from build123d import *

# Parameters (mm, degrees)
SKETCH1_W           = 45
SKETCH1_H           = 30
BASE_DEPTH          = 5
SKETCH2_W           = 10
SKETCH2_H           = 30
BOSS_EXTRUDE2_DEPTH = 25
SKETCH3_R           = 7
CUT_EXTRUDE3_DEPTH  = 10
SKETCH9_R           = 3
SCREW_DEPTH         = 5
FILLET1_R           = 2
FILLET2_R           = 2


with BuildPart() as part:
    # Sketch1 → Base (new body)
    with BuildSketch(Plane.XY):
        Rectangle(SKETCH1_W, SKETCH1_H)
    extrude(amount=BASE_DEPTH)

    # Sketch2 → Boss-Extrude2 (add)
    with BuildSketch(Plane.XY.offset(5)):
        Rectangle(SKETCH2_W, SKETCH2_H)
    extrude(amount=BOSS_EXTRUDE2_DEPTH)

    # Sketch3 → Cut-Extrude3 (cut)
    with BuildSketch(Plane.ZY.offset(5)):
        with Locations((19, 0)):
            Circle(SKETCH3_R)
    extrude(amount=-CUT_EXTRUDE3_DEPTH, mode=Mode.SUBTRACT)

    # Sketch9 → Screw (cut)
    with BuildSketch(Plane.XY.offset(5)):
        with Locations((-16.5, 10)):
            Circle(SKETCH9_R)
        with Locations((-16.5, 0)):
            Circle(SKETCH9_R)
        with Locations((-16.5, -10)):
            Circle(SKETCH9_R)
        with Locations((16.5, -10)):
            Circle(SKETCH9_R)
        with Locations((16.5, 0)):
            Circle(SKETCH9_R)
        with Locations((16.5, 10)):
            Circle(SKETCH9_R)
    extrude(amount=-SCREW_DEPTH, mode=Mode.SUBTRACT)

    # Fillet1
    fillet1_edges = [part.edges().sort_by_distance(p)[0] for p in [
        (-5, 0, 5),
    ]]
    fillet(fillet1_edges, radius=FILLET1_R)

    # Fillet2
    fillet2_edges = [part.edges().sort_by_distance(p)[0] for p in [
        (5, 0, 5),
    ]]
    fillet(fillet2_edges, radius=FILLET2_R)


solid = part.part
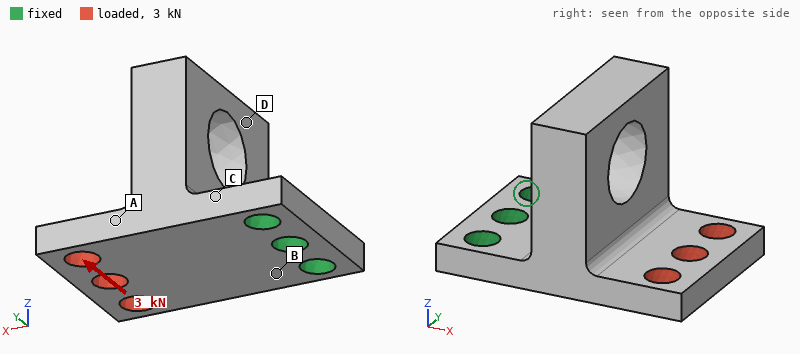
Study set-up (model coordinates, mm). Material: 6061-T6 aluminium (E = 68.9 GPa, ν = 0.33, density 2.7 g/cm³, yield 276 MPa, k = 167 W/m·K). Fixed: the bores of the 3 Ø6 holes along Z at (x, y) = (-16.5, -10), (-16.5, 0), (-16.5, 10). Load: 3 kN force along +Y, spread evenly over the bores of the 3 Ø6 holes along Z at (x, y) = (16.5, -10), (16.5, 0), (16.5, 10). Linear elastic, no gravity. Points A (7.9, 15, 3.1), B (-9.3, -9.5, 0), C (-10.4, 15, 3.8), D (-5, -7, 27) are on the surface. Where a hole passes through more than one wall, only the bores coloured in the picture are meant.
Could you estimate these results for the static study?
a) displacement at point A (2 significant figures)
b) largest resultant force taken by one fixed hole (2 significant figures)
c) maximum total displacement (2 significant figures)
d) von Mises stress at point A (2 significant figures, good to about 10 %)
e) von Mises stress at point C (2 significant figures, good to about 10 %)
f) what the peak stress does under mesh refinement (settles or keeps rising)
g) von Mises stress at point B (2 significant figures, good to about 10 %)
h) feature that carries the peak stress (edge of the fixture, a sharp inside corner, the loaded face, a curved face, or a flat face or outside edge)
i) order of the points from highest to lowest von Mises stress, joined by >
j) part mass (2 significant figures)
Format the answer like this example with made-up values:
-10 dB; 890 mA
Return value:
51 µm; 4.3 kN; 92 µm; 40 MPa; 100 MPa; keeps rising; 76 MPa; edge of the fixture; C > B > A > D; 32 g
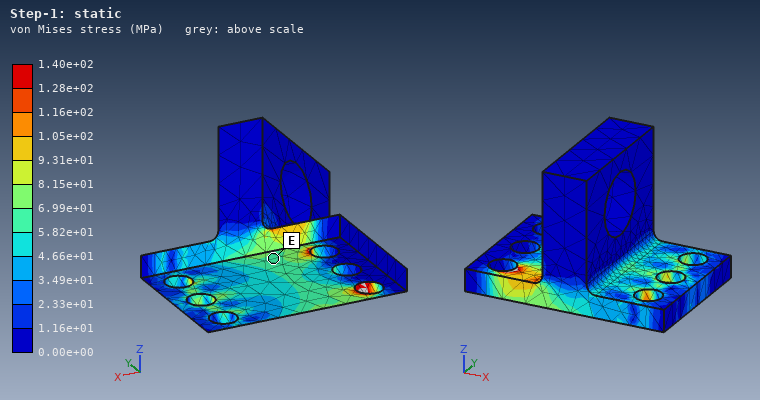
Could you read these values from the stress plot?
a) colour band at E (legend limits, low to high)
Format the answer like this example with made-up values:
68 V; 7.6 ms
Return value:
5.82e+01 to 6.99e+01 MPa
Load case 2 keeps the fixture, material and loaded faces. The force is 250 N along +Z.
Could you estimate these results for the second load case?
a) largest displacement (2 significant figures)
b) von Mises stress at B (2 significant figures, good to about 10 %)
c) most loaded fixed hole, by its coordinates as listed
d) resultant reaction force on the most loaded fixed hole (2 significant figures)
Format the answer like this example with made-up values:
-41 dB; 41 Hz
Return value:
0.11 mm; 49 MPa; (-16.5, 0); 110 N
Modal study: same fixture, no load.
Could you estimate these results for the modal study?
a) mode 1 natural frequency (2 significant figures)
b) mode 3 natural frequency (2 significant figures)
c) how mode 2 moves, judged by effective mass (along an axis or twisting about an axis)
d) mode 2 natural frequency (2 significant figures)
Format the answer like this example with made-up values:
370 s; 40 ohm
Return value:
2300 Hz; 11 kHz; along Y; 5500 Hz
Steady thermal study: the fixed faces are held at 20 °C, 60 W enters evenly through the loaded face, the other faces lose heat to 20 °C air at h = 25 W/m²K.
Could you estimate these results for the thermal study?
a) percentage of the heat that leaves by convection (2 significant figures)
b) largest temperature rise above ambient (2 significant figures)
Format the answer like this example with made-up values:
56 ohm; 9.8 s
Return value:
6.4 %; 74 K
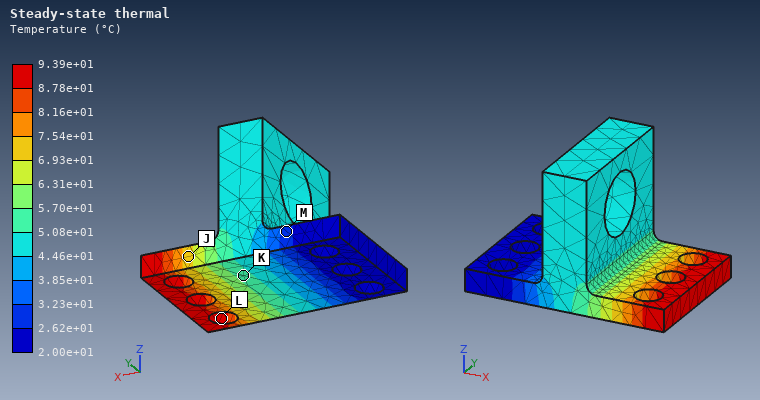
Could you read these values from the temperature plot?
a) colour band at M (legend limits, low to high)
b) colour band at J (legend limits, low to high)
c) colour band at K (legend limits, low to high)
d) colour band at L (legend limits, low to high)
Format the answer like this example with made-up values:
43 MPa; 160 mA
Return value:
2.62e+01 to 3.23e+01 °C; 6.93e+01 to 7.54e+01 °C; 5.08e+01 to 5.70e+01 °C; 8.78e+01 to 9.39e+01 °C
